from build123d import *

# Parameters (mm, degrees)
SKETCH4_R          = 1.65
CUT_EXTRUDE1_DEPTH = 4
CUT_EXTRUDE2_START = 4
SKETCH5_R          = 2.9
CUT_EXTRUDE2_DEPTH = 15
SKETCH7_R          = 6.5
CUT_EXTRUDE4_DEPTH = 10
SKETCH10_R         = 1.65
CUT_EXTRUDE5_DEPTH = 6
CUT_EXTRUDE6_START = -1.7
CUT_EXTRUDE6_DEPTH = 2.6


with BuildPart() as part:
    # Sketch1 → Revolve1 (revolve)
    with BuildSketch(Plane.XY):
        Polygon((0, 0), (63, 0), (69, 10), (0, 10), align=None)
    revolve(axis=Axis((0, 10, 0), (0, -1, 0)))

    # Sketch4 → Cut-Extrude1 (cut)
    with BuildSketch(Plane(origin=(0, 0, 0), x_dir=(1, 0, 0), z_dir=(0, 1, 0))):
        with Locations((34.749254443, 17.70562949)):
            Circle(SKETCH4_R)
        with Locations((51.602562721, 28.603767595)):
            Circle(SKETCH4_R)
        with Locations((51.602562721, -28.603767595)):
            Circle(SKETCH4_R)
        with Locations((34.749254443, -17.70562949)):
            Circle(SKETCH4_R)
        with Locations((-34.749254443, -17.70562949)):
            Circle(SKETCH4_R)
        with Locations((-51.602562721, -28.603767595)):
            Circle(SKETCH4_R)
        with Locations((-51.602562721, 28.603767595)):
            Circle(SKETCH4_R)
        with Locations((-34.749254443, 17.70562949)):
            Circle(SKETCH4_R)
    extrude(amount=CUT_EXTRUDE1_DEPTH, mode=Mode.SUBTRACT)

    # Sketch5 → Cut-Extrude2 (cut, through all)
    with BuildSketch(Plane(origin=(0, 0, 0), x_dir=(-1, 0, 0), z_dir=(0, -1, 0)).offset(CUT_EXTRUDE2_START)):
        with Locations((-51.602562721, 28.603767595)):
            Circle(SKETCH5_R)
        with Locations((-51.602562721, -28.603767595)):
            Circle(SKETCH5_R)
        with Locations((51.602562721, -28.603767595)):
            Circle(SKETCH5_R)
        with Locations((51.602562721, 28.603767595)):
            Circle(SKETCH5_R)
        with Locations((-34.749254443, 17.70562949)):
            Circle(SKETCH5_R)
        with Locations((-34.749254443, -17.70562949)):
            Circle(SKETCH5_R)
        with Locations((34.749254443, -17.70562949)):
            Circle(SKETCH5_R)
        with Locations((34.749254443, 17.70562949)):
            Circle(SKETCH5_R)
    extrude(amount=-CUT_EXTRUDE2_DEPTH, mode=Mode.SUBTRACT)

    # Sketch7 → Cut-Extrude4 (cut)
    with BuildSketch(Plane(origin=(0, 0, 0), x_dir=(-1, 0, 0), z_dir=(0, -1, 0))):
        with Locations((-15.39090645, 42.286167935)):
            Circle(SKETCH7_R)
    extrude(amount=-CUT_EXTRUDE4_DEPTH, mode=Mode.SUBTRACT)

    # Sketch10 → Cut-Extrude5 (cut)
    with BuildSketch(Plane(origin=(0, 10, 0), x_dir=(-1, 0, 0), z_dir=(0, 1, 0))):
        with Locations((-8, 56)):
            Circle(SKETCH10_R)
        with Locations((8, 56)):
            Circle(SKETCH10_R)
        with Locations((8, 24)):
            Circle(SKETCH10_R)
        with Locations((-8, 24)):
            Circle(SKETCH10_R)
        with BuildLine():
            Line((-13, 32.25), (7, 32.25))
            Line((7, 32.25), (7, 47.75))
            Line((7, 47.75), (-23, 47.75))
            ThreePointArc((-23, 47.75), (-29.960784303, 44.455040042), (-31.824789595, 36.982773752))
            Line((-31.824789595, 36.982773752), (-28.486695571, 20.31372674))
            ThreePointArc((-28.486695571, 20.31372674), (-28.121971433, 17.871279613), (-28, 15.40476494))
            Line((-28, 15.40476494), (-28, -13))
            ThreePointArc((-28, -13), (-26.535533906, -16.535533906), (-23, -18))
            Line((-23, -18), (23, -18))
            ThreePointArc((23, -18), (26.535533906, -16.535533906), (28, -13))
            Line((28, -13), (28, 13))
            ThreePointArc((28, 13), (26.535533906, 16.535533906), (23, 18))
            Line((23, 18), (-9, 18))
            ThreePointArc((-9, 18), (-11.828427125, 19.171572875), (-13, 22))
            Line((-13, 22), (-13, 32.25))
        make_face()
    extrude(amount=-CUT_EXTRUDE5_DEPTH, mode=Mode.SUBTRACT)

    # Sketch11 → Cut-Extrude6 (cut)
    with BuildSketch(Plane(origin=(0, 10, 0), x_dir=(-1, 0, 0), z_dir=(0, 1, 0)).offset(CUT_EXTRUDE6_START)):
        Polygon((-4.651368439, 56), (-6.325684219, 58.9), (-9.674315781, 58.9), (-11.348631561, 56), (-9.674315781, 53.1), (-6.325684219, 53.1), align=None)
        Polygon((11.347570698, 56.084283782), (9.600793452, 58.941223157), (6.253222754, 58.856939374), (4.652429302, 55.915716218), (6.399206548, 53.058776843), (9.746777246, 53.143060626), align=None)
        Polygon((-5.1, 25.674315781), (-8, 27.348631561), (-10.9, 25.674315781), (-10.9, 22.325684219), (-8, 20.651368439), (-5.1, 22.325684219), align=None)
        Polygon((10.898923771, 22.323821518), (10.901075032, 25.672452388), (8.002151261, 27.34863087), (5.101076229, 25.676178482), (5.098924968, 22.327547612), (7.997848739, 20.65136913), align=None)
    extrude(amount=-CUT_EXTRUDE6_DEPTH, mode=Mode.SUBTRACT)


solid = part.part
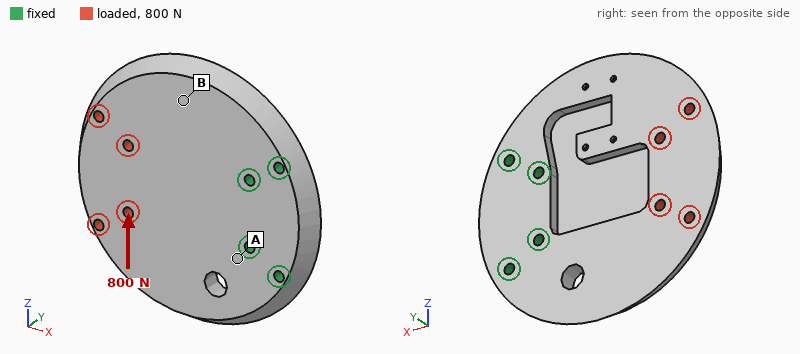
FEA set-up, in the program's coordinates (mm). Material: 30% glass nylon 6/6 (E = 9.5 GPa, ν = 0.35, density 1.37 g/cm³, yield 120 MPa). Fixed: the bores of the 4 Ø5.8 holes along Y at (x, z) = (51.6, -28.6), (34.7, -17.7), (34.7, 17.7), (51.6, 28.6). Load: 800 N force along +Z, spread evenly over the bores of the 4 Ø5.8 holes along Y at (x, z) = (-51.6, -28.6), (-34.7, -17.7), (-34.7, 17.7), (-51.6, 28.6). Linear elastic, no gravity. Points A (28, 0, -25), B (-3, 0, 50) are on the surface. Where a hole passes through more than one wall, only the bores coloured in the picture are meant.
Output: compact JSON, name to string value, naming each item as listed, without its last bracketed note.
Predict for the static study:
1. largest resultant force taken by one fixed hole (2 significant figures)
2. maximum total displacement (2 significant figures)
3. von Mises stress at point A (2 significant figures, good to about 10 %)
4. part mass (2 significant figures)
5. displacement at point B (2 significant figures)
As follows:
{"largest resultant force taken by one fixed hole": "830 N", "maximum total displacement": "0.16 mm", "von Mises stress at point A": "4.7 MPa", "part mass": "160 g", "displacement at point B": "0.073 mm"}
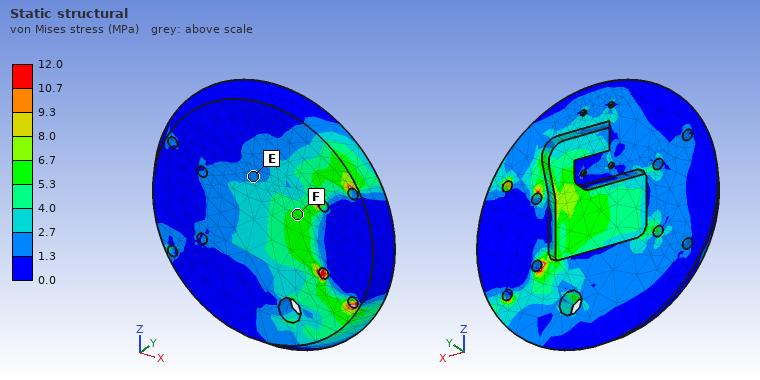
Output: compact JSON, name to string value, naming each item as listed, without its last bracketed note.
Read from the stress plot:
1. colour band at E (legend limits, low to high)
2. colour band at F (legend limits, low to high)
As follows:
{"colour band at E": "1.3 to 2.7 MPa", "colour band at F": "5.3 to 6.7 MPa"}
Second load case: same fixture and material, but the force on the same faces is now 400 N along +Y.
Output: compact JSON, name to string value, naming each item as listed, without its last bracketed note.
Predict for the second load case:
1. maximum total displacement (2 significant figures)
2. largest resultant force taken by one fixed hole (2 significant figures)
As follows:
{"maximum total displacement": "2.2 mm", "largest resultant force taken by one fixed hole": "790 N"}
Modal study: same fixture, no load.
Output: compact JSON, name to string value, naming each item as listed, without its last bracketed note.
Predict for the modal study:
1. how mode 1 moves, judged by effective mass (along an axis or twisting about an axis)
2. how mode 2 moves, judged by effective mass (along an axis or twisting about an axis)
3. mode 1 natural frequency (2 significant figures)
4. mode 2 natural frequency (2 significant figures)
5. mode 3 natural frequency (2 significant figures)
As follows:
{"how mode 1 moves, judged by effective mass": "along Y", "how mode 2 moves, judged by effective mass": "twisting about X", "mode 1 natural frequency": "340 Hz", "mode 2 natural frequency": "690 Hz", "mode 3 natural frequency": "1500 Hz"}
